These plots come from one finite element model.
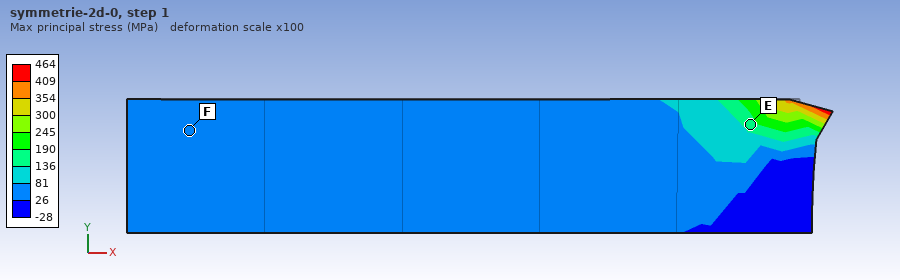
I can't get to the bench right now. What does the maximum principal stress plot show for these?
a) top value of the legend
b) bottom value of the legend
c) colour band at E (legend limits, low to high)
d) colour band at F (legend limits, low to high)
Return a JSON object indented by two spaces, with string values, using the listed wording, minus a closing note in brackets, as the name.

{
  "top value of the legend": "464 MPa",
  "bottom value of the legend": "-28 MPa",
  "colour band at E": "136 to 190 MPa",
  "colour band at F": "26 to 81 MPa"
}
